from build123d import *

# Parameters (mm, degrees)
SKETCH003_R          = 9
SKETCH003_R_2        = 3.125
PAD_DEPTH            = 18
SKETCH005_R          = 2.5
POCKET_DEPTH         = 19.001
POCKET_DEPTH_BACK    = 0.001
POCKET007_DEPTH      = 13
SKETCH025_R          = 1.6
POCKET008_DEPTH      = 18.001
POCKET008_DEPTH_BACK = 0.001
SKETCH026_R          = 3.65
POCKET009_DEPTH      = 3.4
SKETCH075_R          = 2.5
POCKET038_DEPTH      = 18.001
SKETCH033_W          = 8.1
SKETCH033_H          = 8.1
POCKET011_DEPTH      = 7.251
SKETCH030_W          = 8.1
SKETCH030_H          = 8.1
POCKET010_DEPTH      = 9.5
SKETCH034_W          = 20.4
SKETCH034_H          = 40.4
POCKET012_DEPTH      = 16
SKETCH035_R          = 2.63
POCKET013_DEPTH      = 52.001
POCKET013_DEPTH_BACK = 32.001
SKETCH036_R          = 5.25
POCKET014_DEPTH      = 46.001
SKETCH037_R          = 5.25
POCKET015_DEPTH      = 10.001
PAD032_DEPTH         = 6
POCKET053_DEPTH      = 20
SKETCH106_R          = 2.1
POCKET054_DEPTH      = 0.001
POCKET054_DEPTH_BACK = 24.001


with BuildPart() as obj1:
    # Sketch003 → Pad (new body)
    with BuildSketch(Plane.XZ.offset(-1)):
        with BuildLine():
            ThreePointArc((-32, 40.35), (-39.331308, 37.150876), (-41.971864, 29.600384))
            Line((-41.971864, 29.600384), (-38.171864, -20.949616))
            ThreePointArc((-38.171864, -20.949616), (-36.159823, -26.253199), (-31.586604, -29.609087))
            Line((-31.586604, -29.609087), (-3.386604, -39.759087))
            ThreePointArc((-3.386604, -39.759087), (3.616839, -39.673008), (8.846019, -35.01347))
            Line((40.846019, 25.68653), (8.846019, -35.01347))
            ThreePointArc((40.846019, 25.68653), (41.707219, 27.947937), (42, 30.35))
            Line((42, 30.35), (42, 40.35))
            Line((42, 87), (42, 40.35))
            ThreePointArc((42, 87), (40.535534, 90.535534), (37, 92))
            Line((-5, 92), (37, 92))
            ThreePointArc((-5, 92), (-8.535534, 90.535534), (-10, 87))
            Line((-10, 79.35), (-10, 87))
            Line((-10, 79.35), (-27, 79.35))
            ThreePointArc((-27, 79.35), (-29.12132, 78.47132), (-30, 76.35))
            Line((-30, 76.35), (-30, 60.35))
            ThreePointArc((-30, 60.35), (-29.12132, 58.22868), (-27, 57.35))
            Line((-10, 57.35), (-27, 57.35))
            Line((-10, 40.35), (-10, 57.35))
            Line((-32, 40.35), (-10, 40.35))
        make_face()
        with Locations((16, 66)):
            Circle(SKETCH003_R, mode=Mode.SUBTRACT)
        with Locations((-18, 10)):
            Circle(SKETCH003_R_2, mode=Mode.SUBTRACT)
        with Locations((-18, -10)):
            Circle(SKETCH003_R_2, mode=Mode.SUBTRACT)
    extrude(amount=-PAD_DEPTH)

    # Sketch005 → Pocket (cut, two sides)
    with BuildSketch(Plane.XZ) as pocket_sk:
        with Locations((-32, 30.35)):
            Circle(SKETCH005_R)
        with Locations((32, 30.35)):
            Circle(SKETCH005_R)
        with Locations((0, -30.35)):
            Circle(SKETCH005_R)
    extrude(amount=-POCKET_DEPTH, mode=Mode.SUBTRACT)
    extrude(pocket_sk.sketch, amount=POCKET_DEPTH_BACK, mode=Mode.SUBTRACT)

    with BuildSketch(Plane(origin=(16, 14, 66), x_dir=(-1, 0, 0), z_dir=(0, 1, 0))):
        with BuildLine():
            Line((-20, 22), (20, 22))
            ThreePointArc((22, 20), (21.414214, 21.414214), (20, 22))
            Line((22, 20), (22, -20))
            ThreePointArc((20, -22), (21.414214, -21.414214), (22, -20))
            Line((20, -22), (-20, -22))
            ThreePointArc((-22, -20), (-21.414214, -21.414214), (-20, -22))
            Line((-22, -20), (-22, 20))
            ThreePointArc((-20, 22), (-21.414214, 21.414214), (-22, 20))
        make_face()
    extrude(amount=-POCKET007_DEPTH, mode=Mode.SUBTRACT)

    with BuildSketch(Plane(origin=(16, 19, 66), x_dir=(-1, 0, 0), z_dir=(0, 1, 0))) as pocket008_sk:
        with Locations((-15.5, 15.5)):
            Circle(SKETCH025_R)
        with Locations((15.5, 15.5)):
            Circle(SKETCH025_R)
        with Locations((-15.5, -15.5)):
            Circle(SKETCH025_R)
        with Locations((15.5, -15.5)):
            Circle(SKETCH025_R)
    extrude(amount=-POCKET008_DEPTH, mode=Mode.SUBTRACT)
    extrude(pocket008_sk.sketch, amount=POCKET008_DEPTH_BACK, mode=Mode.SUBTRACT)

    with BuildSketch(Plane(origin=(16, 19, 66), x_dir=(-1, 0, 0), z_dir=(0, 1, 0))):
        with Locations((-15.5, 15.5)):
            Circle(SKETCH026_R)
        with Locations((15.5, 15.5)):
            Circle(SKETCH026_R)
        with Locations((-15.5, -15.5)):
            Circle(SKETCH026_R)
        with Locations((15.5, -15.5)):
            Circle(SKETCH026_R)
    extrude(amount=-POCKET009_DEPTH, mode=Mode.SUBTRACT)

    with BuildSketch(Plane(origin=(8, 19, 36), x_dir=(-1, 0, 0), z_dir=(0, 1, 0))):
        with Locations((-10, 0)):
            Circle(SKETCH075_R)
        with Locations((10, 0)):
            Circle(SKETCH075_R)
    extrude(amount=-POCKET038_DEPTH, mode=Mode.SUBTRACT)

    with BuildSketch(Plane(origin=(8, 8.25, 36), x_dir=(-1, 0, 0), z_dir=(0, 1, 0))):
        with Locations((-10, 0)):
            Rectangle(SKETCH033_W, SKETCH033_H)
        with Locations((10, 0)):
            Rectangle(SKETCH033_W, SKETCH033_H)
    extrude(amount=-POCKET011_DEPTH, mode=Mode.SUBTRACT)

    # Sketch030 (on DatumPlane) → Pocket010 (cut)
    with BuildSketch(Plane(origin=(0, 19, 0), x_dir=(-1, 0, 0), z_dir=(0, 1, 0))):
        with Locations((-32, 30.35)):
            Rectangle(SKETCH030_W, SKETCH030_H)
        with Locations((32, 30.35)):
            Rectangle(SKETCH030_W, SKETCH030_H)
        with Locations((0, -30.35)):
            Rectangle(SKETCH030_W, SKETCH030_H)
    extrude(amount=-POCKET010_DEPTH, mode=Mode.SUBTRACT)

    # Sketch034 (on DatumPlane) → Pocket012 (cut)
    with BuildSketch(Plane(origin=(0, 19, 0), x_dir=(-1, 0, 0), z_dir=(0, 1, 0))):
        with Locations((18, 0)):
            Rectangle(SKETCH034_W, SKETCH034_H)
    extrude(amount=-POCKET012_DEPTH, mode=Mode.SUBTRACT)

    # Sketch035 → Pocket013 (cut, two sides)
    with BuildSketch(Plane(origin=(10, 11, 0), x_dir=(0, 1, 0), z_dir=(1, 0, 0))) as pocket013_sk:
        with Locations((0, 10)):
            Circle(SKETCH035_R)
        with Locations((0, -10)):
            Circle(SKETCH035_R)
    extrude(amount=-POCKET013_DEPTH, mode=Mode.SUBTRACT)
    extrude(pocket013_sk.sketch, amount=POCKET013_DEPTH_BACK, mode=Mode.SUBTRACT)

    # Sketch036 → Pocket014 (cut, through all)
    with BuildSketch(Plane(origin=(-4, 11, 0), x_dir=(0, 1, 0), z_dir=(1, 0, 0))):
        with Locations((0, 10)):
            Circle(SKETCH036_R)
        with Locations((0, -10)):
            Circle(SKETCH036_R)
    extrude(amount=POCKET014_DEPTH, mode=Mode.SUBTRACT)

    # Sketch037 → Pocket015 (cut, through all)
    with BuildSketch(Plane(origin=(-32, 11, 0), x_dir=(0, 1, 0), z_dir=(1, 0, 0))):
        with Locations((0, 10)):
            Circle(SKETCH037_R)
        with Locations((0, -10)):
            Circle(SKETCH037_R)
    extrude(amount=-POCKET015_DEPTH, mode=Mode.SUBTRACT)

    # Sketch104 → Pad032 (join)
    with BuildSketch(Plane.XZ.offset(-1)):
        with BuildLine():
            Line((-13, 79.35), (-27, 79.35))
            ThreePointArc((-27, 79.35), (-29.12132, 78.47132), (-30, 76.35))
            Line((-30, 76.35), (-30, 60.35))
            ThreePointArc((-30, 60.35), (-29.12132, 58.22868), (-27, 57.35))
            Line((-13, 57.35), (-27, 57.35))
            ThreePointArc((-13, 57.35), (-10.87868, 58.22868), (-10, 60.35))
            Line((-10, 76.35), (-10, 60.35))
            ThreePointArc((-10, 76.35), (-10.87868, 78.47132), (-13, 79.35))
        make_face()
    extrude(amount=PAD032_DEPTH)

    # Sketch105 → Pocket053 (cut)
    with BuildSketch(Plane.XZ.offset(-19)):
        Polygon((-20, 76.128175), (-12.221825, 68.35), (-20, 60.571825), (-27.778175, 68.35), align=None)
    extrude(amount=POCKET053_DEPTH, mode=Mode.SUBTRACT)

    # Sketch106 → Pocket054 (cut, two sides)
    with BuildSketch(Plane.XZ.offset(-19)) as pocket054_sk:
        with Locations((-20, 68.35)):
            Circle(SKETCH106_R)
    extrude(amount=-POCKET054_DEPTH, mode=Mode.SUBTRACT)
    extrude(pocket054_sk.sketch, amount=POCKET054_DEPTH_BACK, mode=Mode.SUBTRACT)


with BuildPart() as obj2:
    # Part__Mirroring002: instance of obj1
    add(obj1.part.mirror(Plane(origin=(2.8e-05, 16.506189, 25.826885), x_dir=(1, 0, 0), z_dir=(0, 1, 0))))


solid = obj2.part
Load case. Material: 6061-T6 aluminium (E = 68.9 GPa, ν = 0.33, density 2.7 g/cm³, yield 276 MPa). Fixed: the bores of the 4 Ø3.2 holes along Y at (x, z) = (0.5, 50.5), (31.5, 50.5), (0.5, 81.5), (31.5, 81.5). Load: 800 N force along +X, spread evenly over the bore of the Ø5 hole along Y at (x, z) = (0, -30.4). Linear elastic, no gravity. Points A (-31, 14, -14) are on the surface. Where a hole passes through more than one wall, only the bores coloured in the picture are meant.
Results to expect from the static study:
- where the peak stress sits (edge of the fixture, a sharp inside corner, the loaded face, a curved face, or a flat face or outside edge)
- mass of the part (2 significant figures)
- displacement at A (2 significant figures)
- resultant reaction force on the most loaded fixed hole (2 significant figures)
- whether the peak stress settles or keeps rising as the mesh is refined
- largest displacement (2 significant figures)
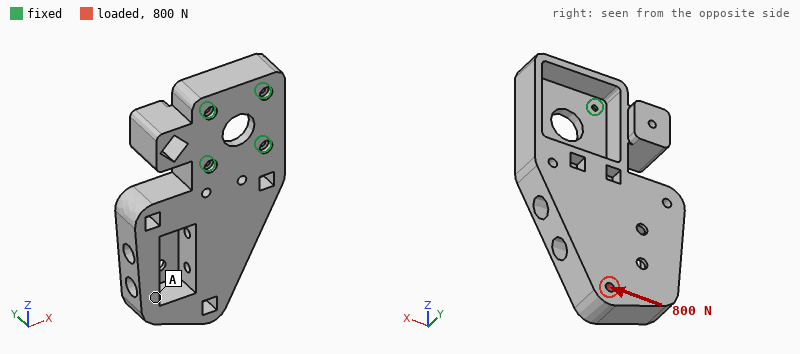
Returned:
edge of the fixture
260 g
41 µm
1.3 kN
keeps rising
51 µm
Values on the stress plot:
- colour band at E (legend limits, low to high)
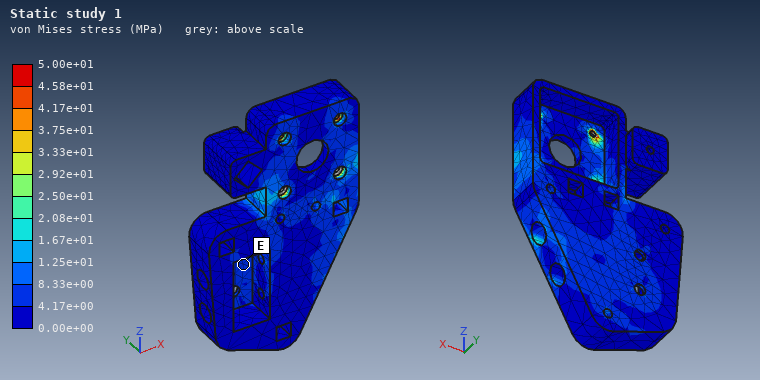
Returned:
4.17e+00 to 8.33e+00 MPa
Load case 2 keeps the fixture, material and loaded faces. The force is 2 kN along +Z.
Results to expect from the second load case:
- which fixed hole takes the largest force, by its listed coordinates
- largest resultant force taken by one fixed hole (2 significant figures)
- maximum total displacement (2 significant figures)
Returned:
(0.5, 50.5)
1.2 kN
0.15 mm
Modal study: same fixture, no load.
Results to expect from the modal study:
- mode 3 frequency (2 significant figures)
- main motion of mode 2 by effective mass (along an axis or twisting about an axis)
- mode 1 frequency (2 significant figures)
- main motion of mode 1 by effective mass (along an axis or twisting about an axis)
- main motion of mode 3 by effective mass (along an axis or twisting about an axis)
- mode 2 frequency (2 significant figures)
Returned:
2400 Hz
twisting about Z
790 Hz
along Y
along X
2300 Hz
